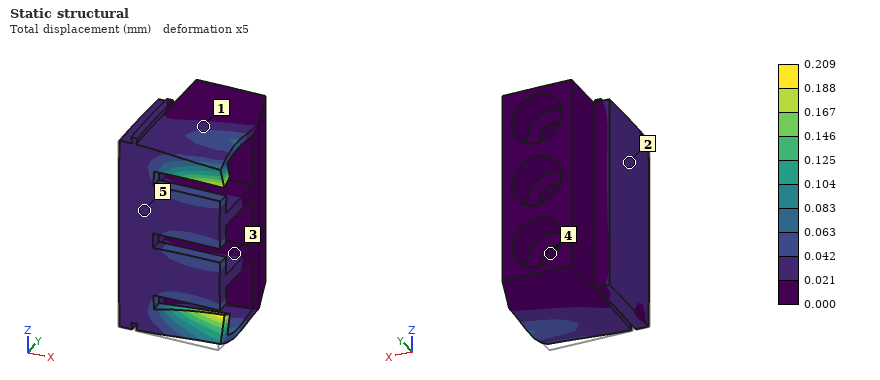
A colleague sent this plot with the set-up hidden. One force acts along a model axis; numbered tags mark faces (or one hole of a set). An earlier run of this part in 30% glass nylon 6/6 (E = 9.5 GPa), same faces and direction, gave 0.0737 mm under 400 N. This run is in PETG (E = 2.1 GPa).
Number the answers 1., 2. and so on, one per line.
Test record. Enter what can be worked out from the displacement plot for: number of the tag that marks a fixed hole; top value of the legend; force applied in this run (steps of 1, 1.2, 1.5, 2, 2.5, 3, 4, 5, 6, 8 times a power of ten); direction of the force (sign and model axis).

1. 4
2. 0.209 mm
3. 250 N
4. +Y
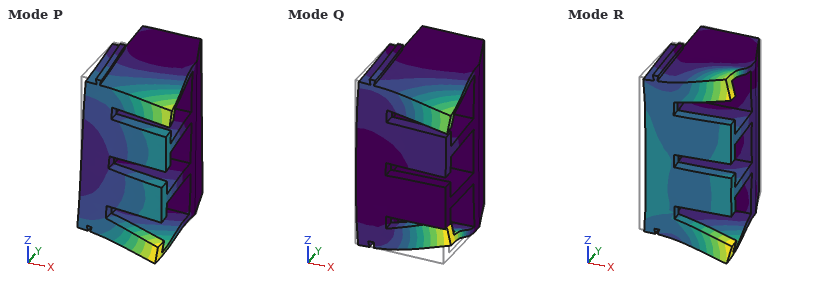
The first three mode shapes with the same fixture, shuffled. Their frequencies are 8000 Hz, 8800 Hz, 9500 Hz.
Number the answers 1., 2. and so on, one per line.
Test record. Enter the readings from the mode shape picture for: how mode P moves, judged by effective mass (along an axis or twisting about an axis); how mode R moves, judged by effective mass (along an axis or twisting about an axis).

1. along Z
2. along X
